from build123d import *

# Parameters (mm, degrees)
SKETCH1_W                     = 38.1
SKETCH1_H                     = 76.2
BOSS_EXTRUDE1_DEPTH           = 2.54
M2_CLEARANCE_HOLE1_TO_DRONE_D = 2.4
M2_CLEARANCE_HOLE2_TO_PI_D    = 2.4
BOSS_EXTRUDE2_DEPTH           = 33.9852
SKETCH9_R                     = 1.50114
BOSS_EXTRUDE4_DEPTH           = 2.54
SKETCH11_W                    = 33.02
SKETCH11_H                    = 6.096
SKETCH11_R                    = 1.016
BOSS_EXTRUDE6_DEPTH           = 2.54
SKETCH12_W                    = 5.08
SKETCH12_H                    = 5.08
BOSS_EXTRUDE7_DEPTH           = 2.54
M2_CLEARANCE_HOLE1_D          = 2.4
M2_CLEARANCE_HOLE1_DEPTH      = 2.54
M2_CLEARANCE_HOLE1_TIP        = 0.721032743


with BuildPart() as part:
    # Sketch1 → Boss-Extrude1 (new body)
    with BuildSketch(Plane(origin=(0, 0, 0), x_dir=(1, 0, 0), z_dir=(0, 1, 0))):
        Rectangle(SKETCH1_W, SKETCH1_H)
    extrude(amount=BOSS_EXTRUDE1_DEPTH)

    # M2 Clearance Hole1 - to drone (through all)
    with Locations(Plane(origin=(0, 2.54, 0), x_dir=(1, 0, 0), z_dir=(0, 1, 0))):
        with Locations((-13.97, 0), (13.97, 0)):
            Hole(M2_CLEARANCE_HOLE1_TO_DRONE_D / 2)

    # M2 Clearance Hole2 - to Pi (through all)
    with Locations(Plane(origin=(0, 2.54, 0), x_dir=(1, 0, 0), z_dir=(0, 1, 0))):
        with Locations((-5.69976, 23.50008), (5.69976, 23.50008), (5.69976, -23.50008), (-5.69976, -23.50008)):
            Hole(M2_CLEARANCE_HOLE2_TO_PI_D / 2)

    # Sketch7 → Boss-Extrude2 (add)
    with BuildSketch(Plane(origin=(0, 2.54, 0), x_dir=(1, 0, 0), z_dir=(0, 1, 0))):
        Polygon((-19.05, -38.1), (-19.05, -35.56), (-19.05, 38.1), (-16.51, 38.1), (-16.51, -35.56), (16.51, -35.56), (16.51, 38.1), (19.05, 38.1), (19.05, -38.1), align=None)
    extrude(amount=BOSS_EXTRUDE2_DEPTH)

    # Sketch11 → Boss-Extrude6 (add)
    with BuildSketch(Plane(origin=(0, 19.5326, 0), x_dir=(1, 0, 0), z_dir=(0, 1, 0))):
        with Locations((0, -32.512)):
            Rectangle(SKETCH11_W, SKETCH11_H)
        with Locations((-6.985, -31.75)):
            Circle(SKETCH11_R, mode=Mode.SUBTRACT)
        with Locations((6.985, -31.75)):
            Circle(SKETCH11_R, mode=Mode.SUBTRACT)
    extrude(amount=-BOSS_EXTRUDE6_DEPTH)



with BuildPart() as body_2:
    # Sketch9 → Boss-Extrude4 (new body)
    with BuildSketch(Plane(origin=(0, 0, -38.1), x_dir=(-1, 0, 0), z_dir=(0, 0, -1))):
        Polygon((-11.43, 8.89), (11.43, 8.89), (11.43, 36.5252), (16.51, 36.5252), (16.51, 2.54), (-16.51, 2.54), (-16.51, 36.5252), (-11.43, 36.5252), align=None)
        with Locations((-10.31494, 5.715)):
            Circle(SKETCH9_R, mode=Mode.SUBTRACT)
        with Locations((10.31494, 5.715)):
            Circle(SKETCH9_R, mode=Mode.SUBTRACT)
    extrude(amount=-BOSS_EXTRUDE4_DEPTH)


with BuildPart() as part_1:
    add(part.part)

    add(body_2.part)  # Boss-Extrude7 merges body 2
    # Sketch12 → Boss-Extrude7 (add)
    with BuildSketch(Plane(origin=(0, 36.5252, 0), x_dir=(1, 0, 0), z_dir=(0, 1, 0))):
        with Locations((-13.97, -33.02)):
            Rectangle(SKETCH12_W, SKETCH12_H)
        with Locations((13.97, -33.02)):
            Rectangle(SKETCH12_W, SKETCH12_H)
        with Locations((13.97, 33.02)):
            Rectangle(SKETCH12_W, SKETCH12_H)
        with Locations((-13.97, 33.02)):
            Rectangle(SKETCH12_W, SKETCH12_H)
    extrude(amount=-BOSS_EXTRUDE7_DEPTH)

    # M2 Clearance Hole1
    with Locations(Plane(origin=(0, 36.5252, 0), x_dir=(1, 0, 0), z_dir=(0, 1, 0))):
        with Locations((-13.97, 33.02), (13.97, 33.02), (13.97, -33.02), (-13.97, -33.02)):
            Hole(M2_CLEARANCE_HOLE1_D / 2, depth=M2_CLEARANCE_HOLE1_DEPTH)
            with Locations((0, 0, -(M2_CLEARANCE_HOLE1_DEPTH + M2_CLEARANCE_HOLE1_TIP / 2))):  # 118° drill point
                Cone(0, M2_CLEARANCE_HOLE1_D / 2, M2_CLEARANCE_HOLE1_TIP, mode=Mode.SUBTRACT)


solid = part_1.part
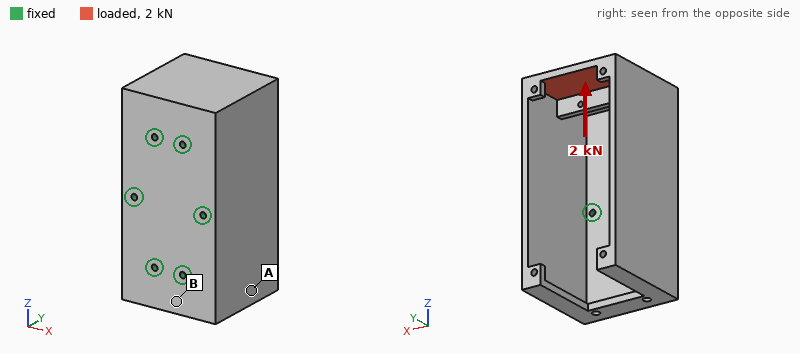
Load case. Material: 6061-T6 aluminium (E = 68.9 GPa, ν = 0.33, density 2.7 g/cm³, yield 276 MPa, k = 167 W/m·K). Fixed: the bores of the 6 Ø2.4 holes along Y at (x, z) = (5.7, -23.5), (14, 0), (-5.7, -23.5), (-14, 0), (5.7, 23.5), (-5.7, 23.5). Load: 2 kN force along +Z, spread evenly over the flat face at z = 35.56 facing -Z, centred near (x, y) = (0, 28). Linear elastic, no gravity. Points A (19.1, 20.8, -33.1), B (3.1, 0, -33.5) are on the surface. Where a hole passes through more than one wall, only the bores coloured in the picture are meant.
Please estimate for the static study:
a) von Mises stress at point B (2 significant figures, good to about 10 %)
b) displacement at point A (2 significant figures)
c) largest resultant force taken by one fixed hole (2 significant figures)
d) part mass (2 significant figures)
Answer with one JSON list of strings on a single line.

["42 MPa", "0.10 mm", "650 N", "68 g"]
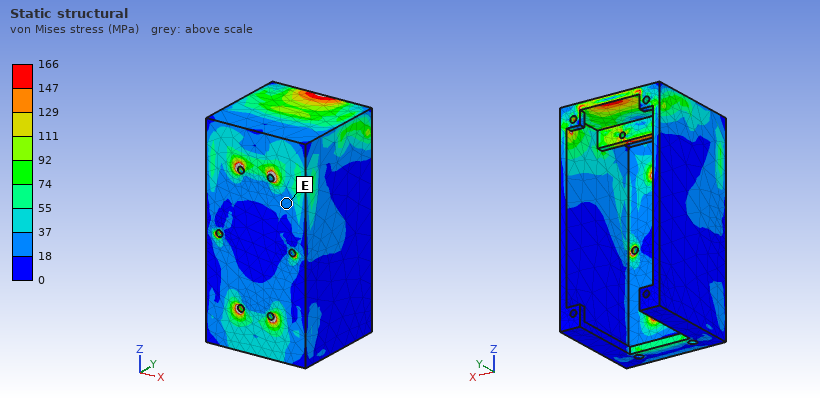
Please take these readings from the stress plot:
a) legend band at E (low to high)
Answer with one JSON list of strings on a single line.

["18 to 37 MPa"]
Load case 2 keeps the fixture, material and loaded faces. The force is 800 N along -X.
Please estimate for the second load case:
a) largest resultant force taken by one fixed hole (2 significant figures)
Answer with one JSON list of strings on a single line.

["800 N"]
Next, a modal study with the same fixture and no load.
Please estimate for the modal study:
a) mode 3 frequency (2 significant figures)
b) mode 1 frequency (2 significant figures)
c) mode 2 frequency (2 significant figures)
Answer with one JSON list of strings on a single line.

["2300 Hz", "2000 Hz", "2300 Hz"]
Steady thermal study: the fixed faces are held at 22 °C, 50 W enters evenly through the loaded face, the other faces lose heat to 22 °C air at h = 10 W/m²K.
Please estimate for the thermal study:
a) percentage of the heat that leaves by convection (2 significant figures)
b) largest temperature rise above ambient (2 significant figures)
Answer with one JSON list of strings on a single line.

["6.2 %", "64 K"]
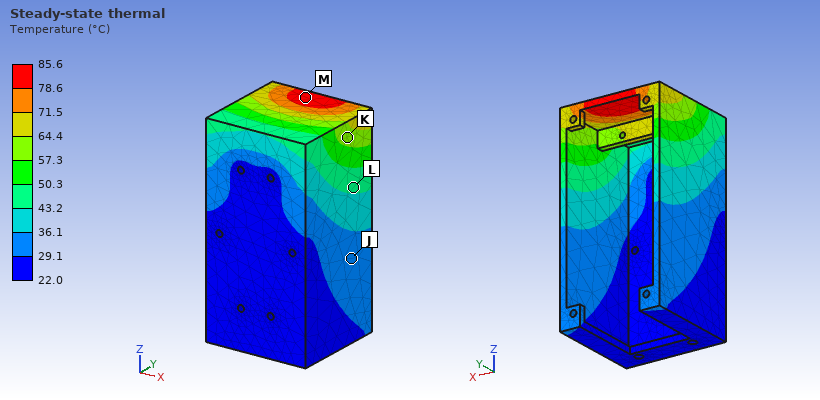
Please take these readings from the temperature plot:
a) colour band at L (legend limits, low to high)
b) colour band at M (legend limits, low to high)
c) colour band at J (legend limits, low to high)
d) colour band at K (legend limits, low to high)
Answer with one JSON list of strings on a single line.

["43.2 to 50.3 °C", "78.6 to 85.6 °C", "29.1 to 36.1 °C", "57.3 to 64.4 °C"]
